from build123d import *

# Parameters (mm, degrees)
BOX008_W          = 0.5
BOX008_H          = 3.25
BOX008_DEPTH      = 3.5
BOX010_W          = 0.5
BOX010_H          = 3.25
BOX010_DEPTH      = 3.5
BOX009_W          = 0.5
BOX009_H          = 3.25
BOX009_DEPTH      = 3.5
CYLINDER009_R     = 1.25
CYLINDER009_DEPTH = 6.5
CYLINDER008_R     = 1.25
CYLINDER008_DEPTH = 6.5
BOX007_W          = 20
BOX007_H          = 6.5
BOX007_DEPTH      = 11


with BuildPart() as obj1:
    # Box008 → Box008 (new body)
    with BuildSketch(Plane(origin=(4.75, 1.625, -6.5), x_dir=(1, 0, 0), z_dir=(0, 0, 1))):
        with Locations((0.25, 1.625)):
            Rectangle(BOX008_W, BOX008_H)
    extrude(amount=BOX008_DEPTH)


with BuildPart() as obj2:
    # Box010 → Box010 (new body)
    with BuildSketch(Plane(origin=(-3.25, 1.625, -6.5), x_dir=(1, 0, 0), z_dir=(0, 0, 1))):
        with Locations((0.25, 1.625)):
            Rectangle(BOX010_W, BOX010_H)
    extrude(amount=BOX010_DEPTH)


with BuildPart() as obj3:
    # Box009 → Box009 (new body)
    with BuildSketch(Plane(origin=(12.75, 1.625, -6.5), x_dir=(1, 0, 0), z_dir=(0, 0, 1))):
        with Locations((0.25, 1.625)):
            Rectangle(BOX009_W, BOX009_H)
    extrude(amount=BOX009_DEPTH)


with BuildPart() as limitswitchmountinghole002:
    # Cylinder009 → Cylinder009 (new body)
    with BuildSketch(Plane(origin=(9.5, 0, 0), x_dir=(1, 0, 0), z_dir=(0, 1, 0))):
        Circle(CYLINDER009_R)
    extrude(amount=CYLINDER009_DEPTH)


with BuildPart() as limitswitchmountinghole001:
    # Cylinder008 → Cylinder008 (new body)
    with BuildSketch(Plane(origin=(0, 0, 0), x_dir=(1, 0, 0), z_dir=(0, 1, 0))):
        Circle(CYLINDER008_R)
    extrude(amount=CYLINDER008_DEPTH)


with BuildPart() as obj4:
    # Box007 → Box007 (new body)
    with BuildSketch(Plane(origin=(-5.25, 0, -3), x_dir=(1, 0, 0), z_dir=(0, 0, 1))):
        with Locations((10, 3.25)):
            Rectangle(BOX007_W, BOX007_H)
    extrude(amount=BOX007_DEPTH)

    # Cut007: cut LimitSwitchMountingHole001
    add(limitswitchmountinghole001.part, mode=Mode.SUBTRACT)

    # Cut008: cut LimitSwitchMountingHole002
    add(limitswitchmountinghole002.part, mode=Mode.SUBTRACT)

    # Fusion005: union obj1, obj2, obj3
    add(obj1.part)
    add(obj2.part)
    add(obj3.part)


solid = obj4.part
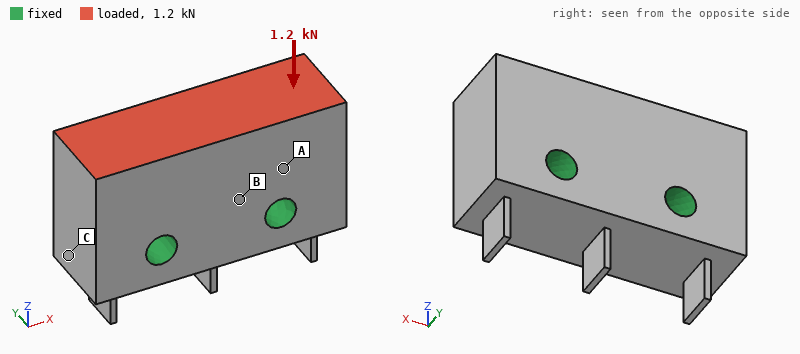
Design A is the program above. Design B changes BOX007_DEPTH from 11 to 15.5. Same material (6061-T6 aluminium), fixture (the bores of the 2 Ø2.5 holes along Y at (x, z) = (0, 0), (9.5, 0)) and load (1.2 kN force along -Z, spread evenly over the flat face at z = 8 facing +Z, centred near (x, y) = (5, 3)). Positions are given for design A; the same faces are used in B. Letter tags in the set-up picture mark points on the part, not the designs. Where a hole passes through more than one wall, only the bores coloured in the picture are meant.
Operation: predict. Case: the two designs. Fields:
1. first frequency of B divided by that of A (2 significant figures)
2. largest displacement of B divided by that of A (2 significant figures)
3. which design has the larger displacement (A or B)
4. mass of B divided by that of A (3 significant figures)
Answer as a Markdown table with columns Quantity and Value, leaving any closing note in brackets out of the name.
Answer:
| Quantity | Value |
|---|---|
| first frequency of B divided by that of A | 0.86 |
| largest displacement of B divided by that of A | 1.1 |
| which design has the larger displacement | B |
| mass of B divided by that of A | 1.42 |
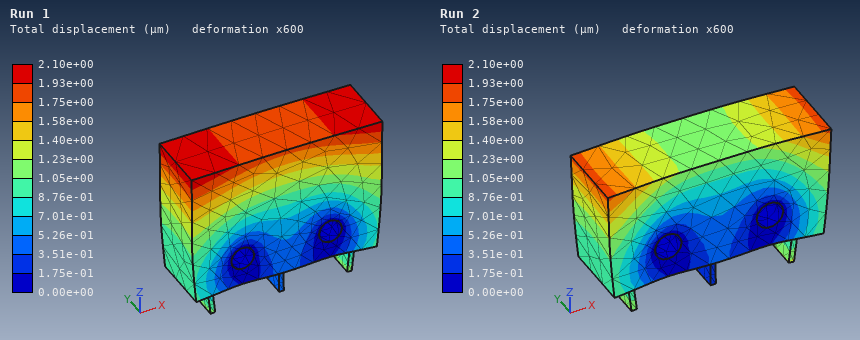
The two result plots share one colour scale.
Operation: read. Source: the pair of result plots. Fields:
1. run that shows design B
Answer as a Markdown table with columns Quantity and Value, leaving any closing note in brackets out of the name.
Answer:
| Quantity | Value |
|---|---|
| run that shows design B | Run 1 |
